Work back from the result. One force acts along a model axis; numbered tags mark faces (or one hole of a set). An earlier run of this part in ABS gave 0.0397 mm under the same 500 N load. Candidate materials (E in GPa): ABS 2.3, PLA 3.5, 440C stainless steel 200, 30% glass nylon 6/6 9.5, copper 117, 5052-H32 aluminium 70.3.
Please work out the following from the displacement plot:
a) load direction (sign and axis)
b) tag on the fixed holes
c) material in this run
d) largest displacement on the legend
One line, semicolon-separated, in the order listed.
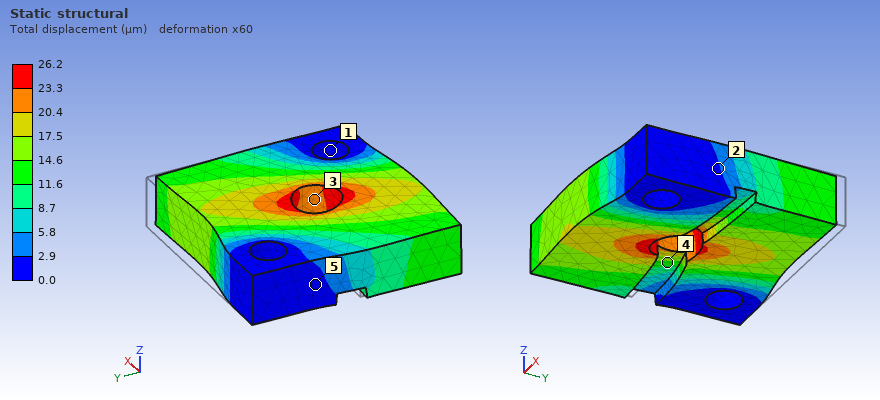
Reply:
-Y; 1; PLA; 26.2 µm
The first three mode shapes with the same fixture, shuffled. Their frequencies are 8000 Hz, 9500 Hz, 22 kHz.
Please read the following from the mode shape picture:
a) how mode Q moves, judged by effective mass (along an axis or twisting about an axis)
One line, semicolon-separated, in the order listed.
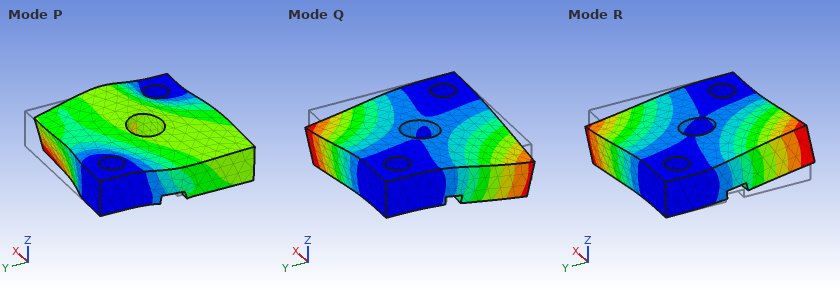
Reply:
along Z
